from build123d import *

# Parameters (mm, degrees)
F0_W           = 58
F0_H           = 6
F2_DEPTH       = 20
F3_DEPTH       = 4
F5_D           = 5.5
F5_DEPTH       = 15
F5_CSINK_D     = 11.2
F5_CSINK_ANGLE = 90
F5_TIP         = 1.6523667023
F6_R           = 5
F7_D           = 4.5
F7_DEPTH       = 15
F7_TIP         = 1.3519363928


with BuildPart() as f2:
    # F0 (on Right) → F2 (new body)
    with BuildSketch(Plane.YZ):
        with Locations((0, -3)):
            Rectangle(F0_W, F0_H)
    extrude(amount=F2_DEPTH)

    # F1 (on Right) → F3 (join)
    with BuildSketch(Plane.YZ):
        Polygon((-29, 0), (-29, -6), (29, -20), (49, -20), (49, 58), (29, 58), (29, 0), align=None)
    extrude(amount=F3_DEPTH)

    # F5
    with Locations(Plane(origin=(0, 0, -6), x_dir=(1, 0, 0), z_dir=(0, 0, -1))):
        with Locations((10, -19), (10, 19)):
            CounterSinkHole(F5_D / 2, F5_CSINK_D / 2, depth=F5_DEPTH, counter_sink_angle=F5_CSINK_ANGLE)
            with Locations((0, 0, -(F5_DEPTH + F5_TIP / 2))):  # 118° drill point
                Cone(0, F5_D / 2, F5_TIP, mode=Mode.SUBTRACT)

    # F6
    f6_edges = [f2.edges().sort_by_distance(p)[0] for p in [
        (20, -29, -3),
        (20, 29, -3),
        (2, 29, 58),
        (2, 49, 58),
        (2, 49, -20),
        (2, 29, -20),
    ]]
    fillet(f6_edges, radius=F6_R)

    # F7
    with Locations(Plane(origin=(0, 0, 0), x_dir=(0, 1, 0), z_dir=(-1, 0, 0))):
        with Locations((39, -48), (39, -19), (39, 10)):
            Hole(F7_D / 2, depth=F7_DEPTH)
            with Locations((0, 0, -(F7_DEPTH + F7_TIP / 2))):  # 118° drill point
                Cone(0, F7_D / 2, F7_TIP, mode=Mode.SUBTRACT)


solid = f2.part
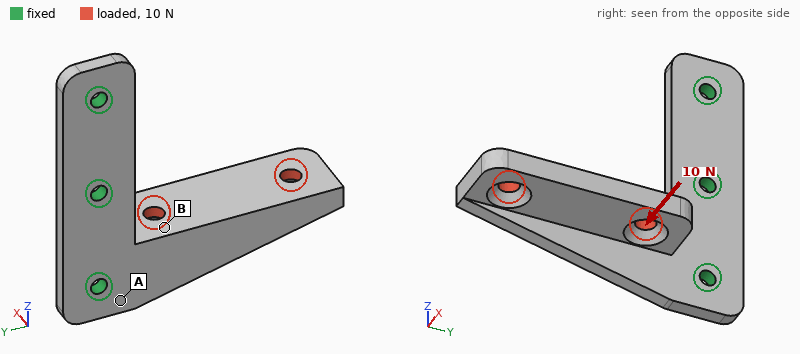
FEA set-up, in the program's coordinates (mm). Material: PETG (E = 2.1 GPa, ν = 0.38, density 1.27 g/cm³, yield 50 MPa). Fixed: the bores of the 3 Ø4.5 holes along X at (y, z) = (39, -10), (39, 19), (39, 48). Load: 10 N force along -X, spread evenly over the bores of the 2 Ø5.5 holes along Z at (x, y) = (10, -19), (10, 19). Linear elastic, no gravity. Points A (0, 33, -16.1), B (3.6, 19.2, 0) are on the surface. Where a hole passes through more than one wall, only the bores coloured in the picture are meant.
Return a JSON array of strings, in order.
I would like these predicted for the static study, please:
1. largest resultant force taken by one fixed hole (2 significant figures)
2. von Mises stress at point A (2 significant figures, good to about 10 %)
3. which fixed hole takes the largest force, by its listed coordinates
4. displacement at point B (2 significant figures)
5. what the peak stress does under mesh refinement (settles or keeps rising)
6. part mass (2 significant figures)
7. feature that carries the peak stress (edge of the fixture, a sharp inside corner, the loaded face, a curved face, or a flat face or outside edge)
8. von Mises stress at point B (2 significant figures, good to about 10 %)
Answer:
["9.0 N", "4.1 MPa", "(39, -10)", "0.25 mm", "keeps rising", "18 g", "edge of the fixture", "1.1 MPa"]
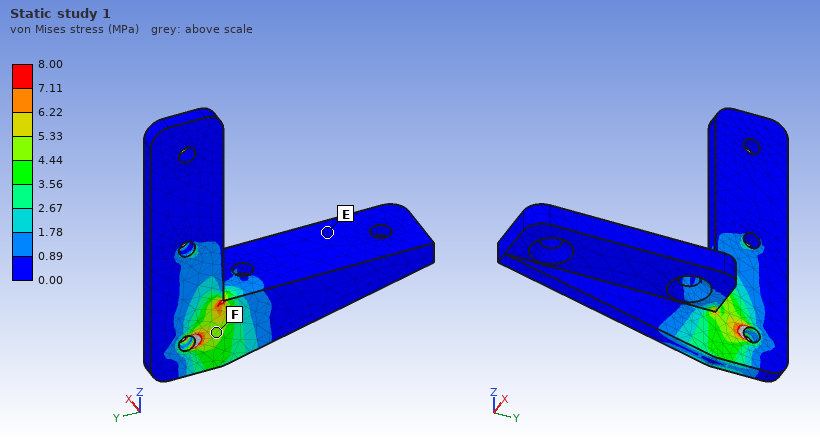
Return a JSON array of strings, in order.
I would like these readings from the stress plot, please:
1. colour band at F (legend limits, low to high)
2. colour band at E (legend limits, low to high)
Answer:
["4.44 to 5.33 MPa", "0.00 to 0.89 MPa"]
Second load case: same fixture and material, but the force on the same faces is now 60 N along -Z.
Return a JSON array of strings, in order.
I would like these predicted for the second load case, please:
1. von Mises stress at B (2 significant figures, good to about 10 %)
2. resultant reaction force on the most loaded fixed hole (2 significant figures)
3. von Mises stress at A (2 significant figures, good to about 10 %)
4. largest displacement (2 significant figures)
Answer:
["5.1 MPa", "82 N", "5.4 MPa", "1.2 mm"]
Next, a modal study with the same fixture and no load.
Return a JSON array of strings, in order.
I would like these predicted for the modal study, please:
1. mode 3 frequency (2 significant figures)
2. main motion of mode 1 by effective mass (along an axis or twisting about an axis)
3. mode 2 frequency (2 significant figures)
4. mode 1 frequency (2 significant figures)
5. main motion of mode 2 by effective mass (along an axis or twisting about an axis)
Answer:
["1100 Hz", "along X", "530 Hz", "190 Hz", "along Z"]
